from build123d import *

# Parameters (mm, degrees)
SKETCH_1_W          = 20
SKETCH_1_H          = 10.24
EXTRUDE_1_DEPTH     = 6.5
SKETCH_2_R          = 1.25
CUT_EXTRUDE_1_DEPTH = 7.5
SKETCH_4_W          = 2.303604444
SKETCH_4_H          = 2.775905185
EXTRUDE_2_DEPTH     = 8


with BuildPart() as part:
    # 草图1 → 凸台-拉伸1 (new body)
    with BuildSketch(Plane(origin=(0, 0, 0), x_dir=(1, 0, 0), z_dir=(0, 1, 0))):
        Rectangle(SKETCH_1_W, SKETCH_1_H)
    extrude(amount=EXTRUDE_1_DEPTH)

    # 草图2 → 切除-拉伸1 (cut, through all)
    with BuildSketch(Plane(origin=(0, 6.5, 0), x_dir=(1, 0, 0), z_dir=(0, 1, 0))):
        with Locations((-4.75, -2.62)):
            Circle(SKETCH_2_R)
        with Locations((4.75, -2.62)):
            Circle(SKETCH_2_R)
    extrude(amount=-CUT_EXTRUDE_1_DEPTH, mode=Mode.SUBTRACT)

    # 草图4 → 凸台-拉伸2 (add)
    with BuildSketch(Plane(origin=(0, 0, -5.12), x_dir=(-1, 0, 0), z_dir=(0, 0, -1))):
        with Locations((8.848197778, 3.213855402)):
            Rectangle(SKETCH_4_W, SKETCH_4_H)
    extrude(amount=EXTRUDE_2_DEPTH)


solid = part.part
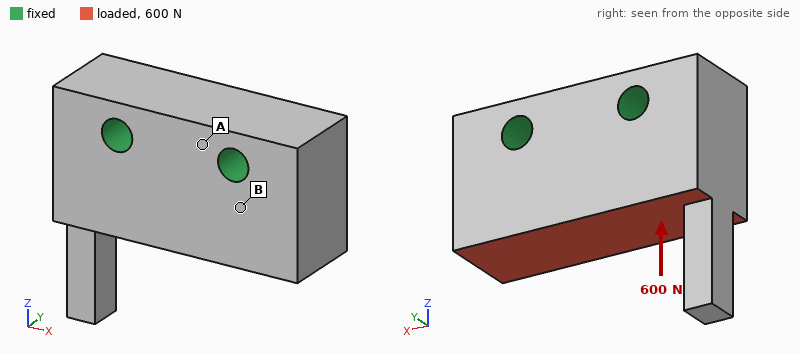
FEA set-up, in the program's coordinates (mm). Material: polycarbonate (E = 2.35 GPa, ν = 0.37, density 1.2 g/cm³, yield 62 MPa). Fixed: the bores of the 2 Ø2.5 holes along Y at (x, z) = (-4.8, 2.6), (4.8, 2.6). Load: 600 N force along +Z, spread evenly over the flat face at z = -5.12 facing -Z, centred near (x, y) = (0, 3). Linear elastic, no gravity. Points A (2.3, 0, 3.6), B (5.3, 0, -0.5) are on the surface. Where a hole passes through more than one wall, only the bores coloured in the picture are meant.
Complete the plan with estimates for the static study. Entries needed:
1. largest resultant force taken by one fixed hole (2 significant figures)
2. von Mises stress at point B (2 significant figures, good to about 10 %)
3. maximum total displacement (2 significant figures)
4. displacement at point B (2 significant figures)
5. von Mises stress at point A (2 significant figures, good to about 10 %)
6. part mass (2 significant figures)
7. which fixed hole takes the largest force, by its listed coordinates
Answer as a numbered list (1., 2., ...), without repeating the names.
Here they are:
1. 320 N
2. 7.3 MPa
3. 31 µm
4. 9.6 µm
5. 3.6 MPa
6. 1.6 g
7. (4.8, 2.6)
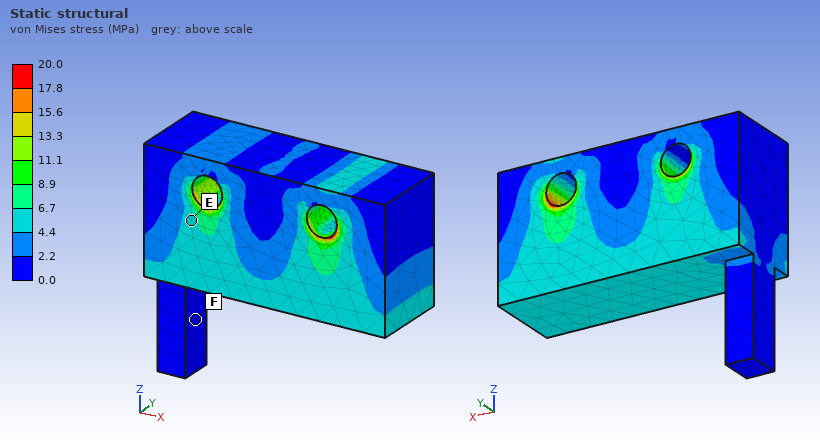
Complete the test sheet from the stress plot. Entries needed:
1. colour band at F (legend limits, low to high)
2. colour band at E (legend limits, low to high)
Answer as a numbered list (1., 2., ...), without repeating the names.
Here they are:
1. 0.0 to 2.2 MPa
2. 4.4 to 6.7 MPa
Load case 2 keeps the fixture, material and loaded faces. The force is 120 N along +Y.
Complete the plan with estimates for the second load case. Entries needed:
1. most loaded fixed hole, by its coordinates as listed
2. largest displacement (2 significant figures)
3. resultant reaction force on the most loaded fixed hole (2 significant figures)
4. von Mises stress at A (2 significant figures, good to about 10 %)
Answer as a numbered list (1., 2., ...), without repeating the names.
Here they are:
1. (4.8, 2.6)
2. 53 µm
3. 63 N
4. 3.2 MPa
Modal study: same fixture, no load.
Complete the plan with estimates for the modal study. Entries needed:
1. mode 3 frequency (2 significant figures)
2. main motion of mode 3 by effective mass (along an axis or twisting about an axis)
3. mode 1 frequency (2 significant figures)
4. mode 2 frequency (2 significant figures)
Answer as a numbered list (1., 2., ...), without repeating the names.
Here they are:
1. 16 kHz
2. along Y
3. 6200 Hz
4. 7000 Hz
